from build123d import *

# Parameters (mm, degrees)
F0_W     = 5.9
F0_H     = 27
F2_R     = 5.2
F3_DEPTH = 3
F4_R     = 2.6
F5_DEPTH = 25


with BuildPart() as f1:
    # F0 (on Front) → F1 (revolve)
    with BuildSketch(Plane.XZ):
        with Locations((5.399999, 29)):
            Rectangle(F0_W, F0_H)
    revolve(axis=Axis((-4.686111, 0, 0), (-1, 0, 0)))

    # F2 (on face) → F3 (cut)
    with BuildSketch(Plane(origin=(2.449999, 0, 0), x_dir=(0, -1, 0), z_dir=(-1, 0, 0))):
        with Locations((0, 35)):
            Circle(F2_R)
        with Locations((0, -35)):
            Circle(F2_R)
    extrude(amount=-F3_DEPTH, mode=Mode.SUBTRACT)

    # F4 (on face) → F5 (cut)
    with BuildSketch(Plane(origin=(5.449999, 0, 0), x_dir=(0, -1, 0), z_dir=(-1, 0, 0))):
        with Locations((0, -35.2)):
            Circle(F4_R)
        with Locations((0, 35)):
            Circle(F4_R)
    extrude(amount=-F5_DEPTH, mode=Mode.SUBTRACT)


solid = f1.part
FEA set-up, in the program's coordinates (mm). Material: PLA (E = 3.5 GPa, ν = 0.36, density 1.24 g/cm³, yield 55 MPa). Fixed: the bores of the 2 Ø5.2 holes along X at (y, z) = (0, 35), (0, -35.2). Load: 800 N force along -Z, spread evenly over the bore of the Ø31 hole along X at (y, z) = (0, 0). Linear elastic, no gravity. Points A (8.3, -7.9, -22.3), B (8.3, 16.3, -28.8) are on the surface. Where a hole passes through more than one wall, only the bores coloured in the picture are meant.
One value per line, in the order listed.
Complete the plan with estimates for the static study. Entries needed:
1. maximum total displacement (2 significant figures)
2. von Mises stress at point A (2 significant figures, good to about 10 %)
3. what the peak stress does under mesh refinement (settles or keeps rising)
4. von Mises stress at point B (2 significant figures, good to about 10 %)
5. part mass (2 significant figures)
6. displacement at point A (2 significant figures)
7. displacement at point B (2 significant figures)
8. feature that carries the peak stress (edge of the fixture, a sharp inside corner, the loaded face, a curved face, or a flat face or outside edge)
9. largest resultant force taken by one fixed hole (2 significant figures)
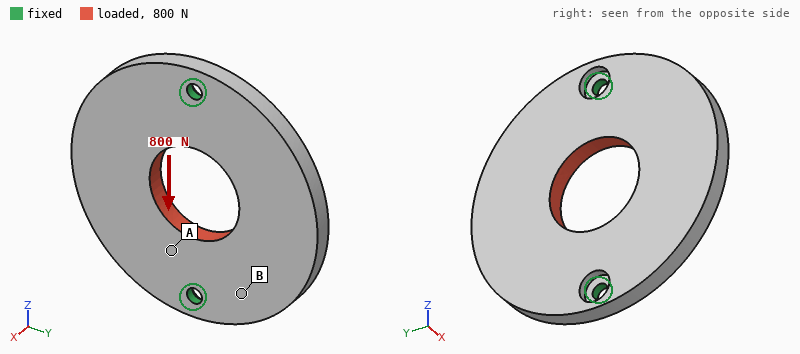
41 µm
3.6 MPa
keeps rising
1.6 MPa
35 g
26 µm
26 µm
edge of the fixture
400 N
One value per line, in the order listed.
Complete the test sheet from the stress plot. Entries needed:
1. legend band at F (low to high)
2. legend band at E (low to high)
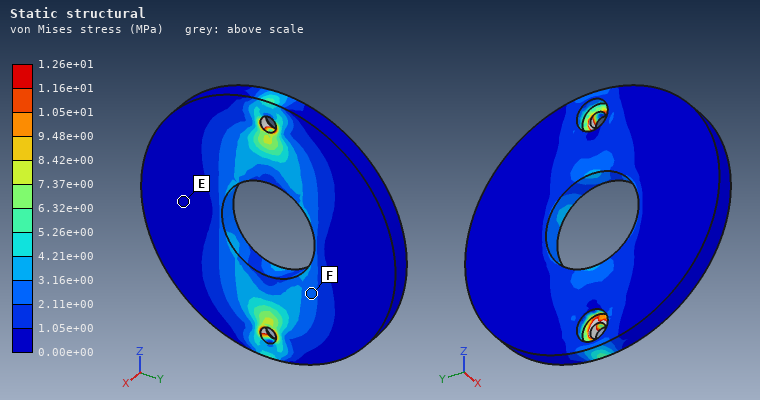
2.11e+00 to 3.16e+00 MPa
0.00e+00 to 1.05e+00 MPa
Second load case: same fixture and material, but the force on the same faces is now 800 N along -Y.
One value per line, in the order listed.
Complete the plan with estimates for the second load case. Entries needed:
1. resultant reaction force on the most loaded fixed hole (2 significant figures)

400 N
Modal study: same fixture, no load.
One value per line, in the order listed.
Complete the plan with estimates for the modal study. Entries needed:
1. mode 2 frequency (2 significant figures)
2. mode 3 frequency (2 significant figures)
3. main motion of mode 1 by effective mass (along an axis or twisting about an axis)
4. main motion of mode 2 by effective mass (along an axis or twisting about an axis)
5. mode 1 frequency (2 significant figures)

760 Hz
1600 Hz
twisting about Z
along X
480 Hz
